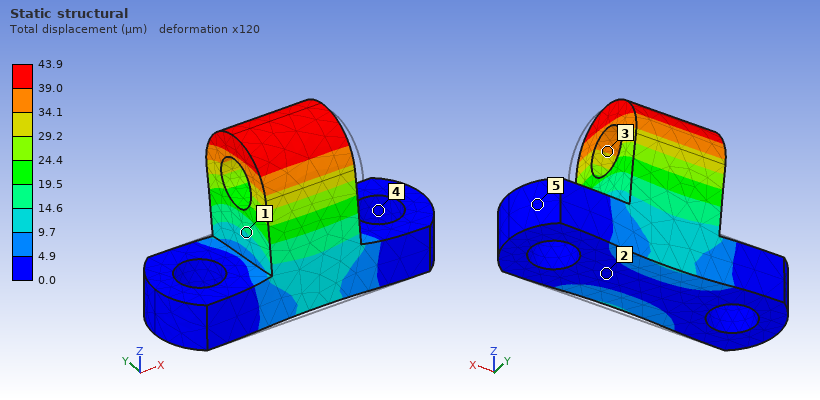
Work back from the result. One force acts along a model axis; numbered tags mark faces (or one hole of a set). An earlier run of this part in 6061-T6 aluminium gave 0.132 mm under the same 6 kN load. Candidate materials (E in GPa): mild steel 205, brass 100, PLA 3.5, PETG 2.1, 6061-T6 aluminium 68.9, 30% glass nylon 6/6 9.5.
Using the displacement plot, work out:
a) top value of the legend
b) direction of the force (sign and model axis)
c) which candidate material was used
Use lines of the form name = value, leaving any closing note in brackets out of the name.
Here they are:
top value of the legend = 43.9 µm
direction of the force = +Y
which candidate material was used = mild steel
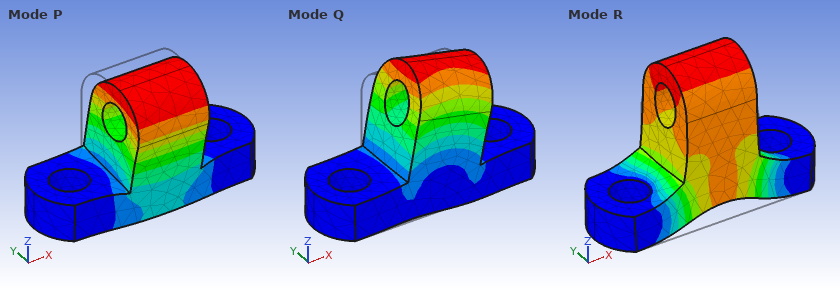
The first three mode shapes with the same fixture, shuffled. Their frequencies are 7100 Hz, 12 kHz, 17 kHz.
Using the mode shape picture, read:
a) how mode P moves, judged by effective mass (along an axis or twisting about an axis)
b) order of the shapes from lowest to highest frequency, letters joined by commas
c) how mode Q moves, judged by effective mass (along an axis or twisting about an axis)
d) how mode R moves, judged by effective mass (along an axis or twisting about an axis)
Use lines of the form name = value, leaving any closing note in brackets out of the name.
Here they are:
how mode P moves, judged by effective mass = along Y
order of the shapes from lowest to highest frequency, letters joined by commas = P, Q, R
how mode Q moves, judged by effective mass = along X
how mode R moves, judged by effective mass = along Z
